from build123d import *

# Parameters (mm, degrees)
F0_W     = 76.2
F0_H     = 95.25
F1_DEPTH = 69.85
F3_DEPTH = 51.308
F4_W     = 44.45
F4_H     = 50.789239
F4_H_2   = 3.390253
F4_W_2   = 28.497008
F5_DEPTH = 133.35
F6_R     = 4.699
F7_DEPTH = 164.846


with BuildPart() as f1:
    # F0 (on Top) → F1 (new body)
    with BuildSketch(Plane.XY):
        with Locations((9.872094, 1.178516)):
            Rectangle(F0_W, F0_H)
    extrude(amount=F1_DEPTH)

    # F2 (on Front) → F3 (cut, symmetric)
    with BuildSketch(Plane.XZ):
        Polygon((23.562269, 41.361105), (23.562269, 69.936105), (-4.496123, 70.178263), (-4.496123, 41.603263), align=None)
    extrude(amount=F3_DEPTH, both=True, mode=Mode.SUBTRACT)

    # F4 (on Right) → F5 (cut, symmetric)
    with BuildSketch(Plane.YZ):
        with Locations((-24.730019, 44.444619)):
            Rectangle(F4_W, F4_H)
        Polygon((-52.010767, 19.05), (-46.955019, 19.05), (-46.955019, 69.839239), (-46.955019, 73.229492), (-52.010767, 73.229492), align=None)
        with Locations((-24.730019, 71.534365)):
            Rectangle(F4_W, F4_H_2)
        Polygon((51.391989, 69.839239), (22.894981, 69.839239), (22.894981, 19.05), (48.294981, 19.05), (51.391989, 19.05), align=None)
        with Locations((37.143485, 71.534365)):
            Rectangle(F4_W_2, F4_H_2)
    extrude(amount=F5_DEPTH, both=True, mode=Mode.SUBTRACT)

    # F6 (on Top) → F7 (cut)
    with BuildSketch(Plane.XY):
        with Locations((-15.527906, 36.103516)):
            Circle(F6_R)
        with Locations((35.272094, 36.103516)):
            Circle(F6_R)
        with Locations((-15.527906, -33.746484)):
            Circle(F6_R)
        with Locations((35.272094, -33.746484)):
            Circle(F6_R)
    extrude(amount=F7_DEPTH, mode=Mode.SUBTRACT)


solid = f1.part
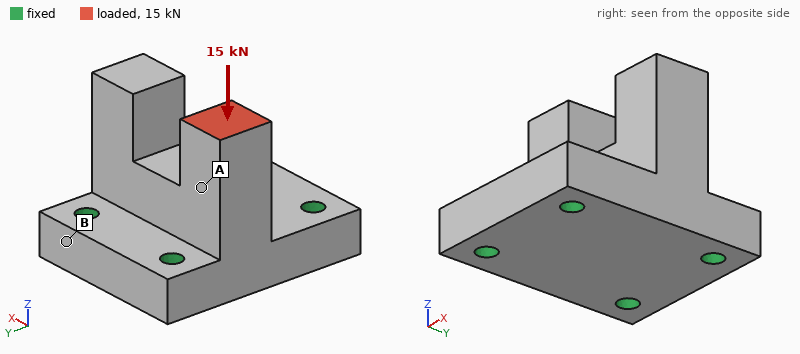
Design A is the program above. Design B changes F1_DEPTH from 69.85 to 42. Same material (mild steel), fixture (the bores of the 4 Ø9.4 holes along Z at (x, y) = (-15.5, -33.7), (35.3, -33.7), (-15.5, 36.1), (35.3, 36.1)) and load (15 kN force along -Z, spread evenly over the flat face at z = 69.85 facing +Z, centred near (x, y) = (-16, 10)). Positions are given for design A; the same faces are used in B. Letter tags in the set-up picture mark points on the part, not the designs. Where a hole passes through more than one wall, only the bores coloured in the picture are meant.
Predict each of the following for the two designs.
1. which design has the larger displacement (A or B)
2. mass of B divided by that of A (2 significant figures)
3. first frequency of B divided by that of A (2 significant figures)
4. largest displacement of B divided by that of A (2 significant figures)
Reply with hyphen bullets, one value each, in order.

- A
- 0.84
- 1.9
- 0.69
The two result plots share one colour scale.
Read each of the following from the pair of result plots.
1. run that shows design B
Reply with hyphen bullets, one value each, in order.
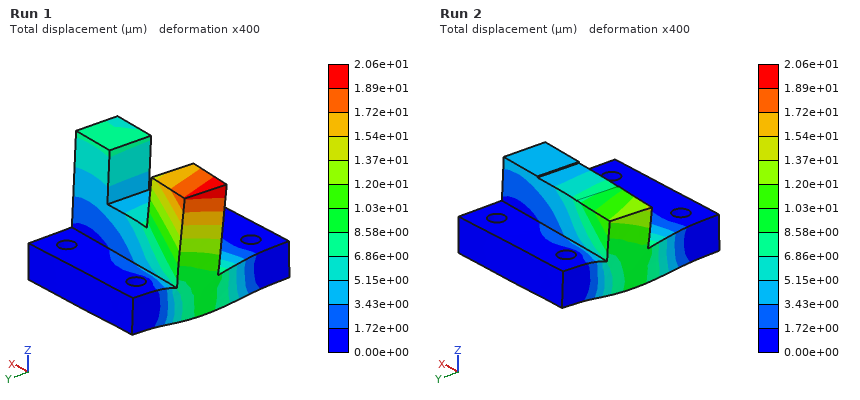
- Run 2
